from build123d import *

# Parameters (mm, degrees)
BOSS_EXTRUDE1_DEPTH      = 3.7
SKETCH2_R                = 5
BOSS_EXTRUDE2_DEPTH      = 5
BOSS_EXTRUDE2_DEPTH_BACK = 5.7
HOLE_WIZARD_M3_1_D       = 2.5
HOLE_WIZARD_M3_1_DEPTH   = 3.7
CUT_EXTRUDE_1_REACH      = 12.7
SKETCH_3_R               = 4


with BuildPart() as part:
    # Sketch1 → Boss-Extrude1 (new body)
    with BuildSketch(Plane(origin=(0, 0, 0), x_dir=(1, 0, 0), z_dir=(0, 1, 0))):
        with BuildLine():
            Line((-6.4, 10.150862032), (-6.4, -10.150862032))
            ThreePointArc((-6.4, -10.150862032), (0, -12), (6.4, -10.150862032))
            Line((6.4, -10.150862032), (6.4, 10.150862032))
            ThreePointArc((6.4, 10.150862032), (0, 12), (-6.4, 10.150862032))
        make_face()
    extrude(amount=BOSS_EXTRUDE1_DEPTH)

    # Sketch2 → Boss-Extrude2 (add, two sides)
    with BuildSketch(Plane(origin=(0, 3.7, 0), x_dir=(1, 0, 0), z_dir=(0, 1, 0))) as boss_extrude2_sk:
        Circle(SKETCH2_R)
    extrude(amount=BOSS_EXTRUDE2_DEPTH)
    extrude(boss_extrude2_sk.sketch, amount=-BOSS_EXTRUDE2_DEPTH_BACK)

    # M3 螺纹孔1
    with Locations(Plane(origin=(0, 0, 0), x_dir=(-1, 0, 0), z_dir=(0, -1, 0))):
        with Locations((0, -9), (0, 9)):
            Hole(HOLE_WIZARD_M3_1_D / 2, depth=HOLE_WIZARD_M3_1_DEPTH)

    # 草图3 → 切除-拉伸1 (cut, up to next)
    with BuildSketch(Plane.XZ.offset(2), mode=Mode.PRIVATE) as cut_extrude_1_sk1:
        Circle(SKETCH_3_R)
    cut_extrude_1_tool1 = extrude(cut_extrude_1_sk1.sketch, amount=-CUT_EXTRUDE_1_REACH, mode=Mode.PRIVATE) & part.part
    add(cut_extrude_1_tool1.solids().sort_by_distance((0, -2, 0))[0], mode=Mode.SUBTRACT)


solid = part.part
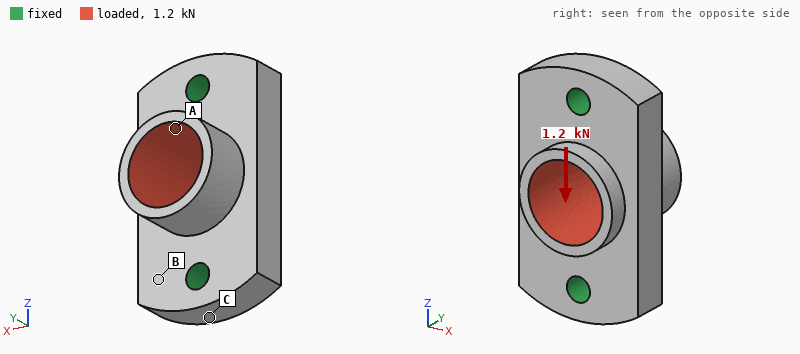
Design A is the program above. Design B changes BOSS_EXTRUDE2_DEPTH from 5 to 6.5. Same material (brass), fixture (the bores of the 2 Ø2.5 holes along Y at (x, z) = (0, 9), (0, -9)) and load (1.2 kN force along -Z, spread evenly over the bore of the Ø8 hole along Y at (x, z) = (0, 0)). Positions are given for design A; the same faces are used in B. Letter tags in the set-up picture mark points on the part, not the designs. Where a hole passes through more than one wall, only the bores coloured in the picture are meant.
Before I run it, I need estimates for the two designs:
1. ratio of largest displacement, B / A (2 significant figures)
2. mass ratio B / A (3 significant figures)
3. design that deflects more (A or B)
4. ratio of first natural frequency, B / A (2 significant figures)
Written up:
1.4
1.04
B
0.89
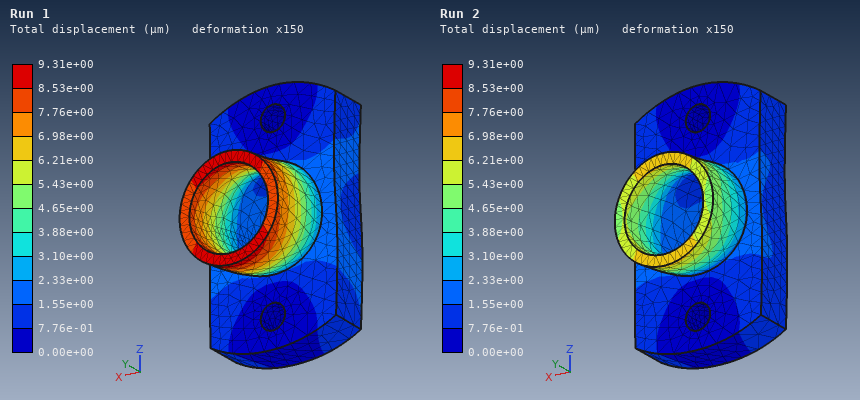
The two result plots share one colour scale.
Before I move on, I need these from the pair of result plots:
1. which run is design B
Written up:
Run 1
